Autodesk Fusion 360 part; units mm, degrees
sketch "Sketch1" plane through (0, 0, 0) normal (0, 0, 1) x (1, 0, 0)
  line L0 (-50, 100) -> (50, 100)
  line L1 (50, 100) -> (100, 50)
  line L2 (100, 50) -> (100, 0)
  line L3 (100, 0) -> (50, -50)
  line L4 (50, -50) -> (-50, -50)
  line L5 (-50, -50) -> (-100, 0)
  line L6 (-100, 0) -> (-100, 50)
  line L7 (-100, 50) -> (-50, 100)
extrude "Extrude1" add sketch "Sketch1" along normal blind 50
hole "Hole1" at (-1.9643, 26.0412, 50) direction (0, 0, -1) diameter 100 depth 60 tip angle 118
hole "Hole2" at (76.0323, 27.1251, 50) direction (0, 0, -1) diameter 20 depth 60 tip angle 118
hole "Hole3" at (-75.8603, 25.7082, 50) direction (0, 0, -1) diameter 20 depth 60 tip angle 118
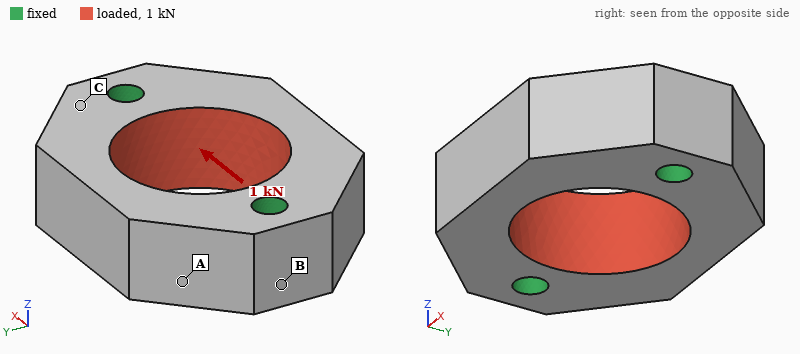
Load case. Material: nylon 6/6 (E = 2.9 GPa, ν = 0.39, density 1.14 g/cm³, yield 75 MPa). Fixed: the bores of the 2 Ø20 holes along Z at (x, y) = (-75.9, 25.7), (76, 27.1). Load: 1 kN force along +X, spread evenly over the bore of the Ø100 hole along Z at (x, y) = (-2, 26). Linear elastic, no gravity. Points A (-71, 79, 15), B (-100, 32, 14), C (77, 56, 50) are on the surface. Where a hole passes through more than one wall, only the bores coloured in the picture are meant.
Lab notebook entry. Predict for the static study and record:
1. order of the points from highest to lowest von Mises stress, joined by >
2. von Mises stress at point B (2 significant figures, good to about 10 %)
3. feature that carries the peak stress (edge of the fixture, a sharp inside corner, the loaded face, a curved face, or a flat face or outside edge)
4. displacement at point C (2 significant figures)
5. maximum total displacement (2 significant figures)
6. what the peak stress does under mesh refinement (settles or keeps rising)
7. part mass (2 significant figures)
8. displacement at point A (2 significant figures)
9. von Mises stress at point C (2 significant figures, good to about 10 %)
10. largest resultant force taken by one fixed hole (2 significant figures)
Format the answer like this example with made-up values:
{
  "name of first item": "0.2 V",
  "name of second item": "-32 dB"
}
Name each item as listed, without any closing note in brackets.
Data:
{
  "order of the points from highest to lowest von Mises stress, joined by >": "B > C > A",
  "von Mises stress at point B": "0.23 MPa",
  "feature that carries the peak stress": "edge of the fixture",
  "displacement at point C": "2.5 µm",
  "maximum total displacement": "7.4 µm",
  "what the peak stress does under mesh refinement": "keeps rising",
  "part mass": "940 g",
  "displacement at point A": "5.5 µm",
  "von Mises stress at point C": "0.11 MPa",
  "largest resultant force taken by one fixed hole": "510 N"
}
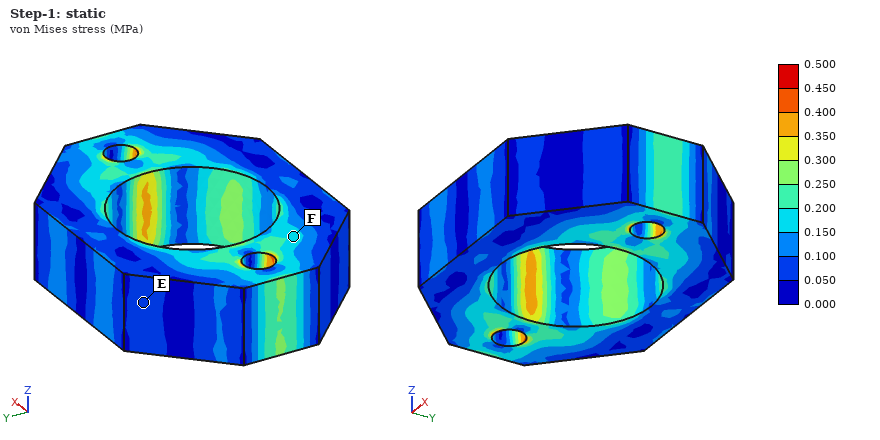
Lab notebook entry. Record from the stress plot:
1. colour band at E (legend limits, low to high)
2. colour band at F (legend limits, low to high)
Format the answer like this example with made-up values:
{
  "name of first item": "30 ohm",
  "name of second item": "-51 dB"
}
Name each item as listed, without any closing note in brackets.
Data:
{
  "colour band at E": "0.050 to 0.100 MPa",
  "colour band at F": "0.150 to 0.200 MPa"
}
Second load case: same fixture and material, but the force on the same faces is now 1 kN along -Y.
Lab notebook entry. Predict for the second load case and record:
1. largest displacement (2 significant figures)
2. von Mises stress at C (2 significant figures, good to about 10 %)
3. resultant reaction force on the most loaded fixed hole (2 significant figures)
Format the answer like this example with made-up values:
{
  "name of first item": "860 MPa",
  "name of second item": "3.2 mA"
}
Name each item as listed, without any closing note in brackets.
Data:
{
  "largest displacement": "8.4 µm",
  "von Mises stress at C": "0.063 MPa",
  "resultant reaction force on the most loaded fixed hole": "510 N"
}
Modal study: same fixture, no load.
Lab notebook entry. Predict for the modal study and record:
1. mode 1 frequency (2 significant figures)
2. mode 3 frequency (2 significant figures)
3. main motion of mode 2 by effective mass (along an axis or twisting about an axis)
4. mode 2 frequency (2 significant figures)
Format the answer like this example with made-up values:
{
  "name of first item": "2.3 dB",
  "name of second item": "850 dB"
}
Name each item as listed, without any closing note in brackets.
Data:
{
  "mode 1 frequency": "1300 Hz",
  "mode 3 frequency": "1900 Hz",
  "main motion of mode 2 by effective mass": "along Z",
  "mode 2 frequency": "1500 Hz"
}
